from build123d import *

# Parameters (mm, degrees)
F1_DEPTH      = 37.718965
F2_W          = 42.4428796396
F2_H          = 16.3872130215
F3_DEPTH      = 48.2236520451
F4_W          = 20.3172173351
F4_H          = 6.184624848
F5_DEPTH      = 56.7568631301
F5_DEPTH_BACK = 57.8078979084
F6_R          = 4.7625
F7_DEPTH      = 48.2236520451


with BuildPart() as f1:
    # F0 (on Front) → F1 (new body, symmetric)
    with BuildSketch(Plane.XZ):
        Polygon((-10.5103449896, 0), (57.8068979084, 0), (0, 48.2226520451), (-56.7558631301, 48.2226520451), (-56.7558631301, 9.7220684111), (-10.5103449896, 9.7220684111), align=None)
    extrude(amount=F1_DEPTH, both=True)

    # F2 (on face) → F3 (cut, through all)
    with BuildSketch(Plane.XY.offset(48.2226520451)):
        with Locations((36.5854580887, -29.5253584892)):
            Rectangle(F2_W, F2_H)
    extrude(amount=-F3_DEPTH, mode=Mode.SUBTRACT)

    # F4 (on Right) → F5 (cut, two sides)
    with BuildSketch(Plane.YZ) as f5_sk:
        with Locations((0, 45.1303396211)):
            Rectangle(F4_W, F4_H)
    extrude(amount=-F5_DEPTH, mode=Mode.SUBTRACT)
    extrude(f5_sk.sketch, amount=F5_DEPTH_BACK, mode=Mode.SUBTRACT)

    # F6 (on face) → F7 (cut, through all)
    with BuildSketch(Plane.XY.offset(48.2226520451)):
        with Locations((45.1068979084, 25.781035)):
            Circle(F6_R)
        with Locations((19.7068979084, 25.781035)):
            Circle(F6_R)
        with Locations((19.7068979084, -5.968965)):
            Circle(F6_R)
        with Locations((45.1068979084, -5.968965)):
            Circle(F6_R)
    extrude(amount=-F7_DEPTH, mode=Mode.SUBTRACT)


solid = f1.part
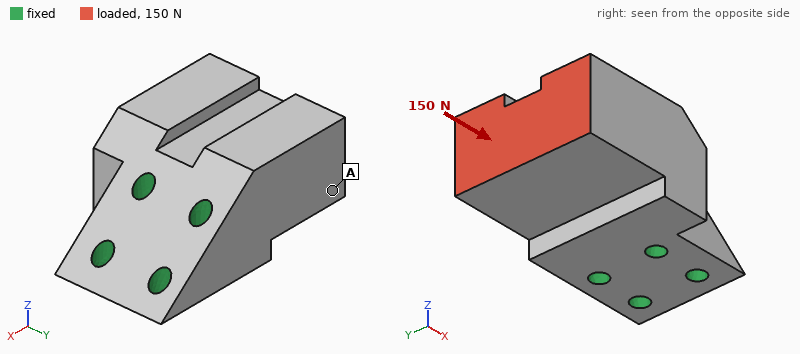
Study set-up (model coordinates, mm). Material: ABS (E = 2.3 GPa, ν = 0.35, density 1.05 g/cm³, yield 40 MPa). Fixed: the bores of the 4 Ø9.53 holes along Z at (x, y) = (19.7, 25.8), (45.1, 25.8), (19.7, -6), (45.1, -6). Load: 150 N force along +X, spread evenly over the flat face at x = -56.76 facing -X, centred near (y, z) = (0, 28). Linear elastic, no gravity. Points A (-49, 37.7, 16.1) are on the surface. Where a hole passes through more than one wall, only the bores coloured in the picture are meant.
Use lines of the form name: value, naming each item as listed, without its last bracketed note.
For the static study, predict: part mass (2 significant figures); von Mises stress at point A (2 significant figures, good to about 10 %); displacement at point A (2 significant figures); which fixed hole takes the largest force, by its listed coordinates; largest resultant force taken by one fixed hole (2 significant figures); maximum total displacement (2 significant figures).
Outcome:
part mass: 260 g
von Mises stress at point A: 0.054 MPa
displacement at point A: 4.0 µm
which fixed hole takes the largest force, by its listed coordinates: (19.7, -6)
largest resultant force taken by one fixed hole: 110 N
maximum total displacement: 7.5 µm
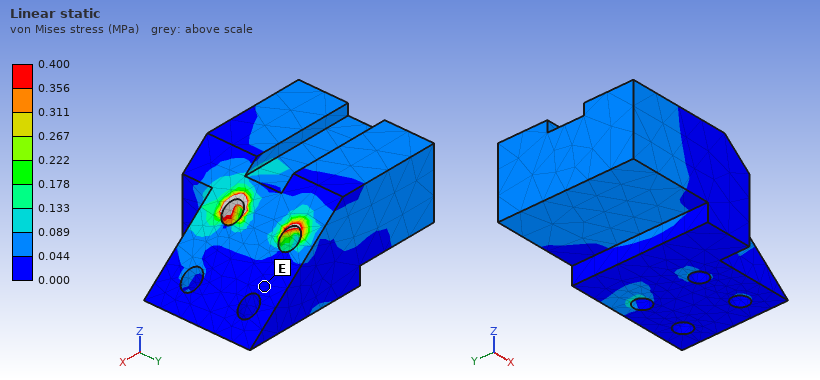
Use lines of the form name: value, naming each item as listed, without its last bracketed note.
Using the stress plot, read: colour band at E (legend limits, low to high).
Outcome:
colour band at E: 0.000 to 0.044 MPa
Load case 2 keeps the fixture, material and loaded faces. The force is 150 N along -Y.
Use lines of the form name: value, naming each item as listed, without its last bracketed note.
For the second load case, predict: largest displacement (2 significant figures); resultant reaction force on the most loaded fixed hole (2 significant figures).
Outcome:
largest displacement: 27 µm
resultant reaction force on the most loaded fixed hole: 290 N
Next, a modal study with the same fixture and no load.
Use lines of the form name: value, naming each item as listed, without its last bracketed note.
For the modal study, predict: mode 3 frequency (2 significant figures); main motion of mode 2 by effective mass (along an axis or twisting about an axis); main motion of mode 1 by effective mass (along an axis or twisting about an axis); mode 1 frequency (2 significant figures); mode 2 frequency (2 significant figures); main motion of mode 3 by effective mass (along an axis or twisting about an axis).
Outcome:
mode 3 frequency: 2000 Hz
main motion of mode 2 by effective mass: along Y
main motion of mode 1 by effective mass: along Z
mode 1 frequency: 1100 Hz
mode 2 frequency: 1400 Hz
main motion of mode 3 by effective mass: twisting about X
